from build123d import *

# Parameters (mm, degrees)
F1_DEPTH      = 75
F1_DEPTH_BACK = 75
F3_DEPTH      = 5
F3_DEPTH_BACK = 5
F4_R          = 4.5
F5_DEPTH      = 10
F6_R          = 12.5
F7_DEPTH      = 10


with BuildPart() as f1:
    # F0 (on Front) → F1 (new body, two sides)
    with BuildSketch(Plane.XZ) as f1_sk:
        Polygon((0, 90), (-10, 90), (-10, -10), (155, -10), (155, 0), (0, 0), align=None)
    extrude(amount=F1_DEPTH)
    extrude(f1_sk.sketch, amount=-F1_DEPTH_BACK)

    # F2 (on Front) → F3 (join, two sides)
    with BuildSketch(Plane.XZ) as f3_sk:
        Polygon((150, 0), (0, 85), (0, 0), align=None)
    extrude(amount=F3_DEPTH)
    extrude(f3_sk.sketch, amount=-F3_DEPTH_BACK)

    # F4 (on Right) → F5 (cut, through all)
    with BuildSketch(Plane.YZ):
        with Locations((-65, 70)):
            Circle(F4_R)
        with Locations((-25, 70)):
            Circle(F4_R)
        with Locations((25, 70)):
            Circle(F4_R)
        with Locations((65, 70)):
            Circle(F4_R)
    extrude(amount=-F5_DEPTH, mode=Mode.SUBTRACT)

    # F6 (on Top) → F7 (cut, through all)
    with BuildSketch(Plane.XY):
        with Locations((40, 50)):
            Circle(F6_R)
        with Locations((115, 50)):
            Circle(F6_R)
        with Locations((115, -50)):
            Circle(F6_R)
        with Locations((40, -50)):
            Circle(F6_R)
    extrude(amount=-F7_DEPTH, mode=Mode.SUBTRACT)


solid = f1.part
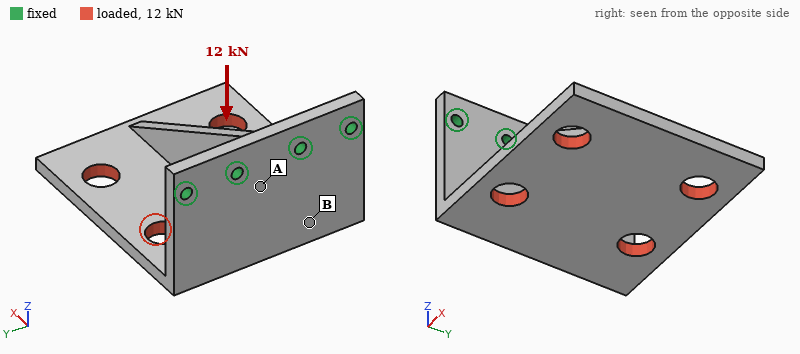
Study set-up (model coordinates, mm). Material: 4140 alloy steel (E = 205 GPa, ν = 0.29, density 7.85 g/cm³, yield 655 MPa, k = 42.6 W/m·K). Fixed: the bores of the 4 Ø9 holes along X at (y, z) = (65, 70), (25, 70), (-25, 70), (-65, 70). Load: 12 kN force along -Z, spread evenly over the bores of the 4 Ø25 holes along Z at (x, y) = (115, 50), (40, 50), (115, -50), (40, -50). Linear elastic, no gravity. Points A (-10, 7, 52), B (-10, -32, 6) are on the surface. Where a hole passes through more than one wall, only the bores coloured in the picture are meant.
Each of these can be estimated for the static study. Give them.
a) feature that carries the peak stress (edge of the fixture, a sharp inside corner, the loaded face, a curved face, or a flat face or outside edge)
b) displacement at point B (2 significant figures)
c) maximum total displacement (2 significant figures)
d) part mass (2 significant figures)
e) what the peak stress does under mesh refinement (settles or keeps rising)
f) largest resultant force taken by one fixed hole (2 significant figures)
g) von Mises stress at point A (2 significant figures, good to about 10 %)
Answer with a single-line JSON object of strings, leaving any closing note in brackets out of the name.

{"feature that carries the peak stress": "edge of the fixture", "displacement at point B": "0.34 mm", "maximum total displacement": "1.2 mm", "part mass": "3.3 kg", "what the peak stress does under mesh refinement": "keeps rising", "largest resultant force taken by one fixed hole": "6.7 kN", "von Mises stress at point A": "120 MPa"}
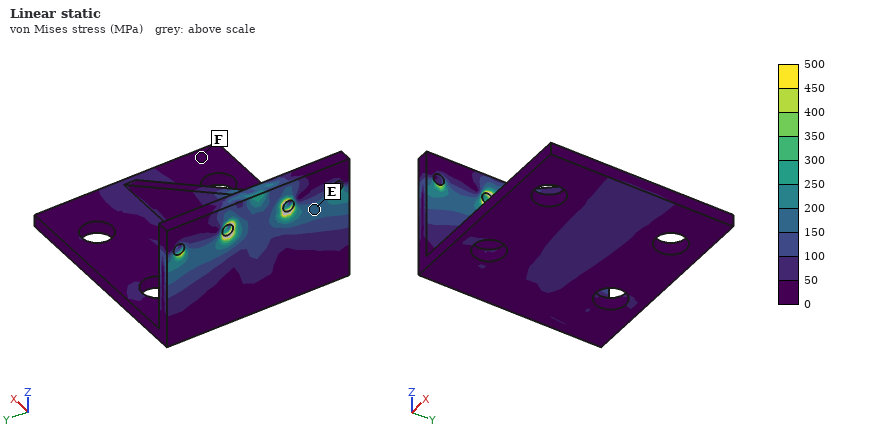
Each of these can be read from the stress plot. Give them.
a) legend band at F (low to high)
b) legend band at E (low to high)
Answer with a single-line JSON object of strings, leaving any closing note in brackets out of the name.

{"legend band at F": "0 to 50 MPa", "legend band at E": "150 to 200 MPa"}
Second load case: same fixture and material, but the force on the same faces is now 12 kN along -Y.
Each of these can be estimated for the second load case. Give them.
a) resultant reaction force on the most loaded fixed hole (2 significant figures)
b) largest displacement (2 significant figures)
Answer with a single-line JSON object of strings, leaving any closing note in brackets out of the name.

{"resultant reaction force on the most loaded fixed hole": "8.1 kN", "largest displacement": "1.0 mm"}
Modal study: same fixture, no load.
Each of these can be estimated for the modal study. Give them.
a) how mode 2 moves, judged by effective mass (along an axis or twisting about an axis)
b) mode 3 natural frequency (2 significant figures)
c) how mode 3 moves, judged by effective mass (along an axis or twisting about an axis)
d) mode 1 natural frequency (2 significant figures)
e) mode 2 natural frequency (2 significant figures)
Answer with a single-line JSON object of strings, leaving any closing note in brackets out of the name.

{"how mode 2 moves, judged by effective mass": "along Y", "mode 3 natural frequency": "900 Hz", "how mode 3 moves, judged by effective mass": "twisting about X", "mode 1 natural frequency": "390 Hz", "mode 2 natural frequency": "460 Hz"}
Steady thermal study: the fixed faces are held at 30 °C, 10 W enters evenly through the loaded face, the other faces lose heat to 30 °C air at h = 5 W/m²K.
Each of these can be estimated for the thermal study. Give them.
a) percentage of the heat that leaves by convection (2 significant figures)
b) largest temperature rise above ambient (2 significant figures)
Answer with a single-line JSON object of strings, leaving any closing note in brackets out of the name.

{"percentage of the heat that leaves by convection": "35 %", "largest temperature rise above ambient": "14 K"}
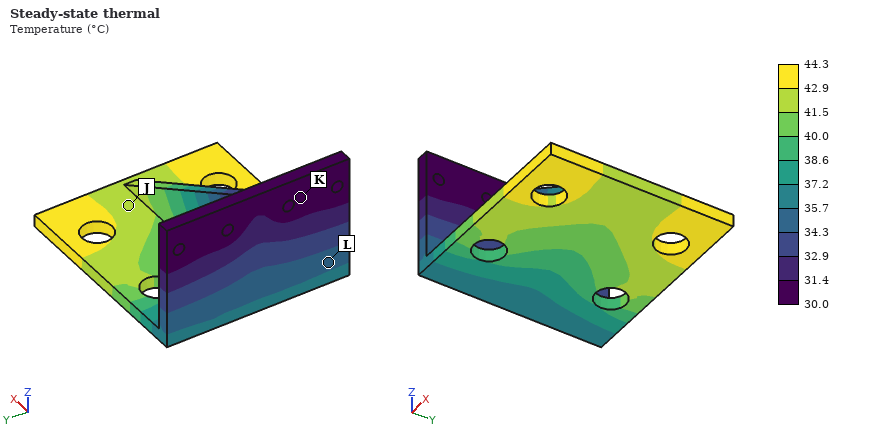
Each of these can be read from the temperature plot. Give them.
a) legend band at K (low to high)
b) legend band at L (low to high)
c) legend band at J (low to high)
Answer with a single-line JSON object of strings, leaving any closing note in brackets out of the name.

{"legend band at K": "30.0 to 31.4 °C", "legend band at L": "34.3 to 35.7 °C", "legend band at J": "41.5 to 42.9 °C"}
